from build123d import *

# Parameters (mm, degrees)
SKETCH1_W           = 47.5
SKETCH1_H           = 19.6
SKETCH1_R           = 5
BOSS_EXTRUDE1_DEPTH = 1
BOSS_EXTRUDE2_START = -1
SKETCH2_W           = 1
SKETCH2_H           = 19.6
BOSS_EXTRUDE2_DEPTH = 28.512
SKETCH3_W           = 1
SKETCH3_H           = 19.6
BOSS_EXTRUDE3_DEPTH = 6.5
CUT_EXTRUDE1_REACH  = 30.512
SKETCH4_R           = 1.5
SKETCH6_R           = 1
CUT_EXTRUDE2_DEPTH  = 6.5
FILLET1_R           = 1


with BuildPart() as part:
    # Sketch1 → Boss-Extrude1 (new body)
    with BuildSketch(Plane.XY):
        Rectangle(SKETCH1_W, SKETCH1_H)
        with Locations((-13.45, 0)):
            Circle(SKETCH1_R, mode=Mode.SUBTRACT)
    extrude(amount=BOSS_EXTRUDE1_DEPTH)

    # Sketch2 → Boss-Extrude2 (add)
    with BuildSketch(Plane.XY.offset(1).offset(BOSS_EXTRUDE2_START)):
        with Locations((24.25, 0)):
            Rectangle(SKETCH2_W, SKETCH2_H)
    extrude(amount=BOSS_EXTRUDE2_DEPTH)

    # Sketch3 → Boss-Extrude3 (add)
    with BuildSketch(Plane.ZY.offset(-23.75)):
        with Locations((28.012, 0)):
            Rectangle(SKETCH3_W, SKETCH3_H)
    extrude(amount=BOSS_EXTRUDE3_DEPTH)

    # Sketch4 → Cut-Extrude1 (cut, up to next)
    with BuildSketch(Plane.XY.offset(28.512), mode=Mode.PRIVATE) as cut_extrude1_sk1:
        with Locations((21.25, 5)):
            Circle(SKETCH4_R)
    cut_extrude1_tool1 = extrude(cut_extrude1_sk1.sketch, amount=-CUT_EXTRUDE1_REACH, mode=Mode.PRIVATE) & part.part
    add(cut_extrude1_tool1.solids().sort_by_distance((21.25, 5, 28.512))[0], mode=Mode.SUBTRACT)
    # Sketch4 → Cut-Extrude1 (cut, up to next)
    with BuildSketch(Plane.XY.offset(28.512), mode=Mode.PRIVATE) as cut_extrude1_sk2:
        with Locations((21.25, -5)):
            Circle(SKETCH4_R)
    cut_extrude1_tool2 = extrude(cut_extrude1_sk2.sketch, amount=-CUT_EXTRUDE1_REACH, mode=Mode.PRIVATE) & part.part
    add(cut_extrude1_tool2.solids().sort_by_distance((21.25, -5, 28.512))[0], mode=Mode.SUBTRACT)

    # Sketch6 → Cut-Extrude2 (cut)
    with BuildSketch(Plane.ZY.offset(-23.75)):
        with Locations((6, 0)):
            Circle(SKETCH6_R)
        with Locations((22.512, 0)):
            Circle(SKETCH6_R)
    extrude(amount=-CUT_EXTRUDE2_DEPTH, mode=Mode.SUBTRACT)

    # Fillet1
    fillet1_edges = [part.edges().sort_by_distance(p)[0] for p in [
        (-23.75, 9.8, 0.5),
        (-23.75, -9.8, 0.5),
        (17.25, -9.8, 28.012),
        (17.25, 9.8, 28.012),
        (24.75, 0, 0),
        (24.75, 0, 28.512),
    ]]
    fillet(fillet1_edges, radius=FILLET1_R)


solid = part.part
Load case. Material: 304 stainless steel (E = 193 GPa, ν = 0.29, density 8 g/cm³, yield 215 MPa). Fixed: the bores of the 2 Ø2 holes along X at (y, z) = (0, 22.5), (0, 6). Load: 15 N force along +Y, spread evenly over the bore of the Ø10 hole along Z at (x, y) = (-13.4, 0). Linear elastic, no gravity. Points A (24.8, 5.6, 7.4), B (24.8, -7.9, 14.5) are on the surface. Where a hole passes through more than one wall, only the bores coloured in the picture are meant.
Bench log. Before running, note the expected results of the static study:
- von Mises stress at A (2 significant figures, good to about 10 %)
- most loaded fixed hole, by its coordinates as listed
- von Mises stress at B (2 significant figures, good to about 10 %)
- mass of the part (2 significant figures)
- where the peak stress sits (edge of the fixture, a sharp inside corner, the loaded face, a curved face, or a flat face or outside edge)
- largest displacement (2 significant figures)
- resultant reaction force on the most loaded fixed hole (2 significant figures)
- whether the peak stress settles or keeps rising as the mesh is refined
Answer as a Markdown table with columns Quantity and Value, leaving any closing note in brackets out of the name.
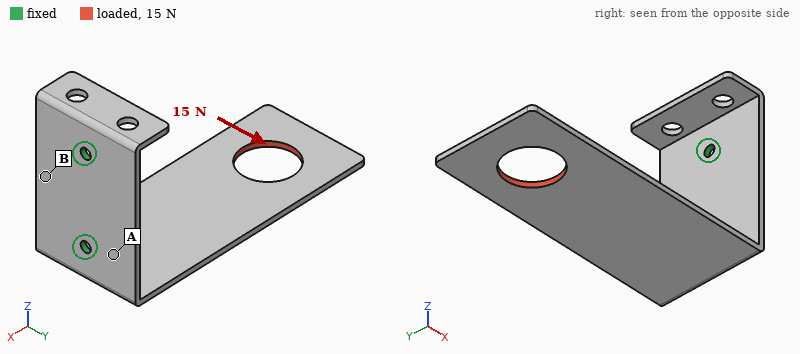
| Quantity | Value |
|---|---|
| von Mises stress at A | 72 MPa |
| most loaded fixed hole, by its coordinates as listed | (0, 6) |
| von Mises stress at B | 30 MPa |
| mass of the part | 12 g |
| where the peak stress sits | edge of the fixture |
| largest displacement | 0.29 mm |
| resultant reaction force on the most loaded fixed hole | 19 N |
| whether the peak stress settles or keeps rising as the mesh is refined | keeps rising |
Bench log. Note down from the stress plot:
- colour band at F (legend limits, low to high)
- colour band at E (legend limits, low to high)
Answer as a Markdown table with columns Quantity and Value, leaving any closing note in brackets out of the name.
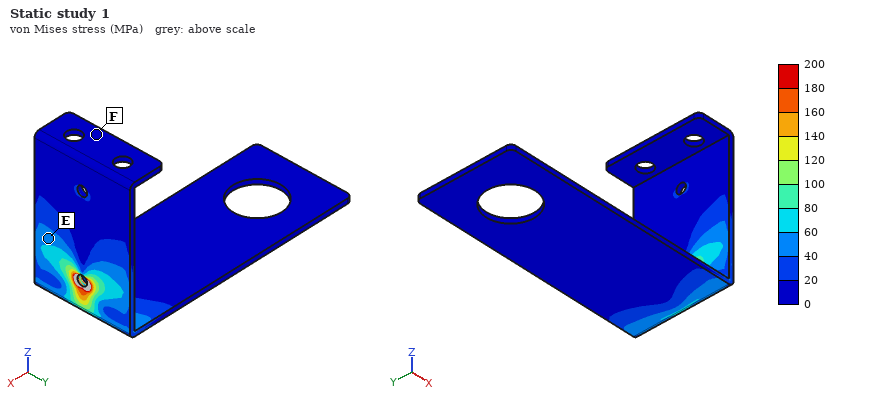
| Quantity | Value |
|---|---|
| colour band at F | 0 to 20 MPa |
| colour band at E | 40 to 60 MPa |
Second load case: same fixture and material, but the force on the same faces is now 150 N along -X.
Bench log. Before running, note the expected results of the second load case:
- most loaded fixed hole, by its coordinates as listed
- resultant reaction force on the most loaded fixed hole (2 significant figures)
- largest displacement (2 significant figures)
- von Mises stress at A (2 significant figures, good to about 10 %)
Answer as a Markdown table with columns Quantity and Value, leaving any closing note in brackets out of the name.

| Quantity | Value |
|---|---|
| most loaded fixed hole, by its coordinates as listed | (0, 6) |
| resultant reaction force on the most loaded fixed hole | 160 N |
| largest displacement | 0.41 mm |
| von Mises stress at A | 73 MPa |
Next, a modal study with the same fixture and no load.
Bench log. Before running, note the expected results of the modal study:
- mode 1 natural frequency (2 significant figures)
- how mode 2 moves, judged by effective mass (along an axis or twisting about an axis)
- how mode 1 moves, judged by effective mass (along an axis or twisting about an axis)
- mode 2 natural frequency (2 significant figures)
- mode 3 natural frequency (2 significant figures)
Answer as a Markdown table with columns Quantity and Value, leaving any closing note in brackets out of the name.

| Quantity | Value |
|---|---|
| mode 1 natural frequency | 310 Hz |
| how mode 2 moves, judged by effective mass | along Y |
| how mode 1 moves, judged by effective mass | along Z |
| mode 2 natural frequency | 680 Hz |
| mode 3 natural frequency | 1700 Hz |
